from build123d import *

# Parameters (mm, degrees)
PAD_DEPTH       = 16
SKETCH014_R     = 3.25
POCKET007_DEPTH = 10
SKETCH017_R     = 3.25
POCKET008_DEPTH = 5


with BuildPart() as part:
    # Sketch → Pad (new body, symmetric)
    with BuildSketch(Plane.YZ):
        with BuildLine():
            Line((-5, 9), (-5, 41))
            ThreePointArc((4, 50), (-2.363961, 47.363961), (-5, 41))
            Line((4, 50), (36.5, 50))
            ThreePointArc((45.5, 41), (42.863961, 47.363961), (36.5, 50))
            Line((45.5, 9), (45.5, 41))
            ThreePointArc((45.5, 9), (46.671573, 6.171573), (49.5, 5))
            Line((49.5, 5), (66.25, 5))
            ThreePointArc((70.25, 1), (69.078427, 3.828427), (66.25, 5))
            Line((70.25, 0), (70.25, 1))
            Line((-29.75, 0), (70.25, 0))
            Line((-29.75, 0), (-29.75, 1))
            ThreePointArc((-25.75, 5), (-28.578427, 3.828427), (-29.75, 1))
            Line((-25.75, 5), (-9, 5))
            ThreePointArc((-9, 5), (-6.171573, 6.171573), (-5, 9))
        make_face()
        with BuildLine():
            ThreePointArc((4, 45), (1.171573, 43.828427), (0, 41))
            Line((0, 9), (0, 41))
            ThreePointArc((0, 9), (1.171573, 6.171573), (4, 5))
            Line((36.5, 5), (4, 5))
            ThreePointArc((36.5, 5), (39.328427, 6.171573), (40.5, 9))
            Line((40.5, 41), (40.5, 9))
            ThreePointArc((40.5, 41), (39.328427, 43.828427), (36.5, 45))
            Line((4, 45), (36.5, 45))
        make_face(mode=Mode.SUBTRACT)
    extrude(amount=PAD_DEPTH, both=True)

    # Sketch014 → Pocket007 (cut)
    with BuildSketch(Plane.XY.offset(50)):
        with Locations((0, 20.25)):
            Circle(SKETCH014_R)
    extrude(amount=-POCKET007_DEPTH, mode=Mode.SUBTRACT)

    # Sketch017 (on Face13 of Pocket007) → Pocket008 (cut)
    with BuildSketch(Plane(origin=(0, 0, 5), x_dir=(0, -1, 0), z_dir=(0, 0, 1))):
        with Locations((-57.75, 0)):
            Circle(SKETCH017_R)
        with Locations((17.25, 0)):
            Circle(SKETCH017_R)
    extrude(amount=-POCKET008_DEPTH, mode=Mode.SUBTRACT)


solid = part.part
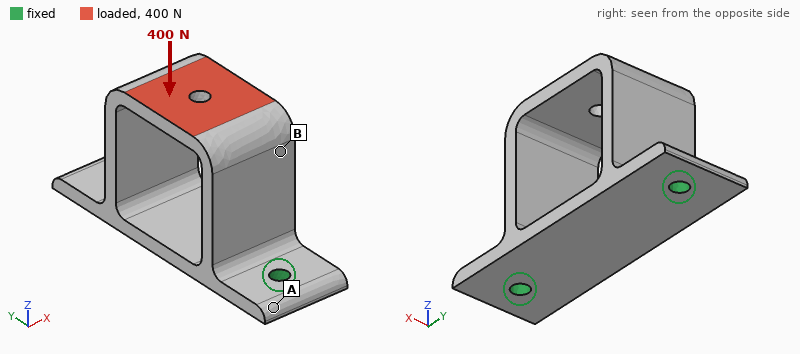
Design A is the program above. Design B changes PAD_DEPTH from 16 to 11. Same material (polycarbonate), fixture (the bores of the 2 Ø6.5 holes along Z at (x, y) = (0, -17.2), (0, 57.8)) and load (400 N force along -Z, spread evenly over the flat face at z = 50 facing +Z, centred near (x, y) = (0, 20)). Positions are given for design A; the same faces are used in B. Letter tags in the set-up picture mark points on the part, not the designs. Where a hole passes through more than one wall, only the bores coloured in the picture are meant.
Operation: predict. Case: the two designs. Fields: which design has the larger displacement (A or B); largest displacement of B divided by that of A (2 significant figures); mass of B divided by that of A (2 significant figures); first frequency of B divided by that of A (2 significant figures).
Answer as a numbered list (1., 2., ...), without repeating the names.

1. B
2. 1.4
3. 0.68
4. 1.0
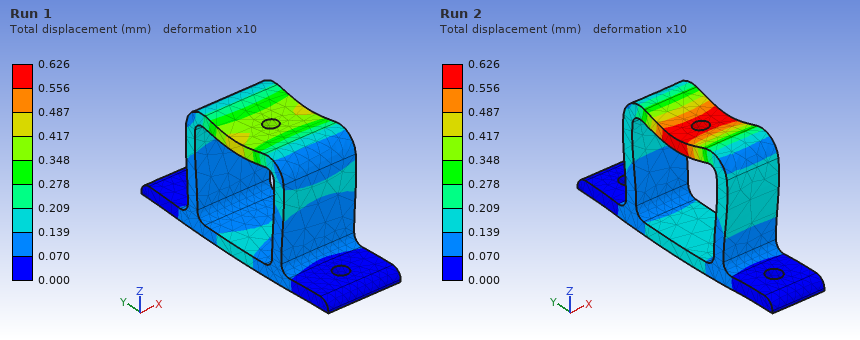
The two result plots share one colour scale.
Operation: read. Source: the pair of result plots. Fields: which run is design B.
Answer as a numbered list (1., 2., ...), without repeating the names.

1. Run 2
